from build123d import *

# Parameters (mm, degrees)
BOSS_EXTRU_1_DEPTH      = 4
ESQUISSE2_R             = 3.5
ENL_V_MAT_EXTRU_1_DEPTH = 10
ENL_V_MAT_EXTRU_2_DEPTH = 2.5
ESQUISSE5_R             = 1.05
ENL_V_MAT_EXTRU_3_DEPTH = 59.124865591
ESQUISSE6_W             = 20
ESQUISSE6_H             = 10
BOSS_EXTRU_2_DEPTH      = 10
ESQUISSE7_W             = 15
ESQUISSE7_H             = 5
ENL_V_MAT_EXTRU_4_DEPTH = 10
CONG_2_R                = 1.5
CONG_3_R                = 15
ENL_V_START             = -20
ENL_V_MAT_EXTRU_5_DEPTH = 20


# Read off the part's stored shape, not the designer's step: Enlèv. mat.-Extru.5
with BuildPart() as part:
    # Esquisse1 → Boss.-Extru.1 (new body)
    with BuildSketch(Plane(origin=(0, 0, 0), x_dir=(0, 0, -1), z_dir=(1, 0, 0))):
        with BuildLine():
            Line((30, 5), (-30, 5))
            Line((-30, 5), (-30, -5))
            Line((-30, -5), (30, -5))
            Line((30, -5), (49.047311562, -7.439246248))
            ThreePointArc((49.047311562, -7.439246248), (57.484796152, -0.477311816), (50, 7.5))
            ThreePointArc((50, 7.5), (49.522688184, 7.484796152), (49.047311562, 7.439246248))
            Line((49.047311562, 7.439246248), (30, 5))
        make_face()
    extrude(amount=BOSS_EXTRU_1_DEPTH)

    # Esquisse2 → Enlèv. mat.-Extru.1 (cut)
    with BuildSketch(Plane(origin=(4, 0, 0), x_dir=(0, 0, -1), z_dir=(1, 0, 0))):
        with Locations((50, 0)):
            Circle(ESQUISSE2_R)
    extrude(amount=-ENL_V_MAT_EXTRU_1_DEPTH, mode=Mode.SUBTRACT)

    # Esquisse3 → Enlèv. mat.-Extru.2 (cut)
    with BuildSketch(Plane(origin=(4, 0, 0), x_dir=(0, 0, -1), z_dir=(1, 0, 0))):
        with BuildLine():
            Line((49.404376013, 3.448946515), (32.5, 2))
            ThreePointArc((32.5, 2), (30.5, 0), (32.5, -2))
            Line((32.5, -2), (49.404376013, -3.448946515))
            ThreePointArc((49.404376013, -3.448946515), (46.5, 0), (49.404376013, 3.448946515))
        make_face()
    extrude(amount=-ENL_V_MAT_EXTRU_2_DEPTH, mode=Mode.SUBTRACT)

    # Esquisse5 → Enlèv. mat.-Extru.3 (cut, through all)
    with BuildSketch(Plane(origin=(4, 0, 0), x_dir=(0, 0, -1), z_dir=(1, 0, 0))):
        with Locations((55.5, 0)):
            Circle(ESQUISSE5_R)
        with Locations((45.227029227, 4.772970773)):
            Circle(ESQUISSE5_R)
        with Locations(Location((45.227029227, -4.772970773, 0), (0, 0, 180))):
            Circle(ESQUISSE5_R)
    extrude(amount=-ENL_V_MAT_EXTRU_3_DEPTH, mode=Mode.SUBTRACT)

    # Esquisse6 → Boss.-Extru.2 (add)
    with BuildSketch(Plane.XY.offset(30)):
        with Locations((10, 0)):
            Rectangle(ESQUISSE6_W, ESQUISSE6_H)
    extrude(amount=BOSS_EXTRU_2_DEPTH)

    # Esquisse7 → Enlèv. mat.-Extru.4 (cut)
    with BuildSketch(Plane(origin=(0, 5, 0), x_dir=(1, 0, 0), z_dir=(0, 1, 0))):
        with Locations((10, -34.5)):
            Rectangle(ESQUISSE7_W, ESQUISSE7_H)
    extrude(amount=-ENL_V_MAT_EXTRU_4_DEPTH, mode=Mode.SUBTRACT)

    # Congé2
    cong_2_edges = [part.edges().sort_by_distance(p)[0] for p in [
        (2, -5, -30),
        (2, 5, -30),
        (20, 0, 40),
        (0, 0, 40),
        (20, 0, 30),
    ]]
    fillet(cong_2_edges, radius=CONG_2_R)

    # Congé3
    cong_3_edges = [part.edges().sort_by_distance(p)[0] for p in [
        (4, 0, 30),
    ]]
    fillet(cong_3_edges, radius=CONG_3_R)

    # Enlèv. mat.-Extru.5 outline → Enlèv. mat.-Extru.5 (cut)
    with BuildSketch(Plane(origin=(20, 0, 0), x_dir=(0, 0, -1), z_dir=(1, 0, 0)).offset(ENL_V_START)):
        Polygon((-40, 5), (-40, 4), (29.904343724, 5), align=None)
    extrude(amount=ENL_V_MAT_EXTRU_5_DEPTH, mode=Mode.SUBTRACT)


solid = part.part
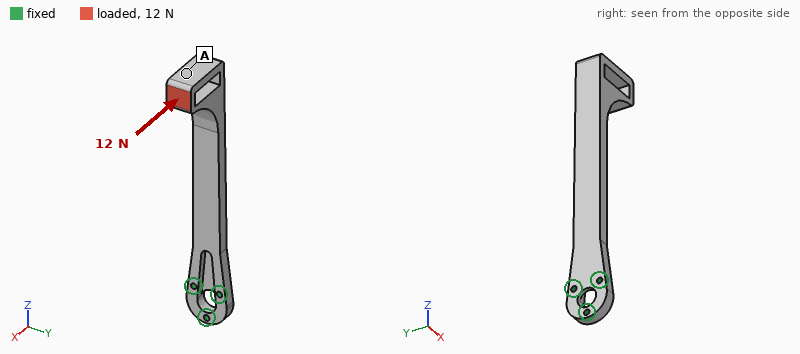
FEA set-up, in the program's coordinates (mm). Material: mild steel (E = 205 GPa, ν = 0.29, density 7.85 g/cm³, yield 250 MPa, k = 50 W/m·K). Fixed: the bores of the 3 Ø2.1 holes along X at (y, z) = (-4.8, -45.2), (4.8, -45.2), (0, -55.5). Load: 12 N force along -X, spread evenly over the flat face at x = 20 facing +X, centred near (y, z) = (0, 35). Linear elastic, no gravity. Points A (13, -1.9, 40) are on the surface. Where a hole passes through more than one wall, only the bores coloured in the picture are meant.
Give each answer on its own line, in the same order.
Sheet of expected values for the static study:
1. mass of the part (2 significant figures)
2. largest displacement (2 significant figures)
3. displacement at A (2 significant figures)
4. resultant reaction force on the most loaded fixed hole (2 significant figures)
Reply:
38 g
0.23 mm
0.22 mm
25 N
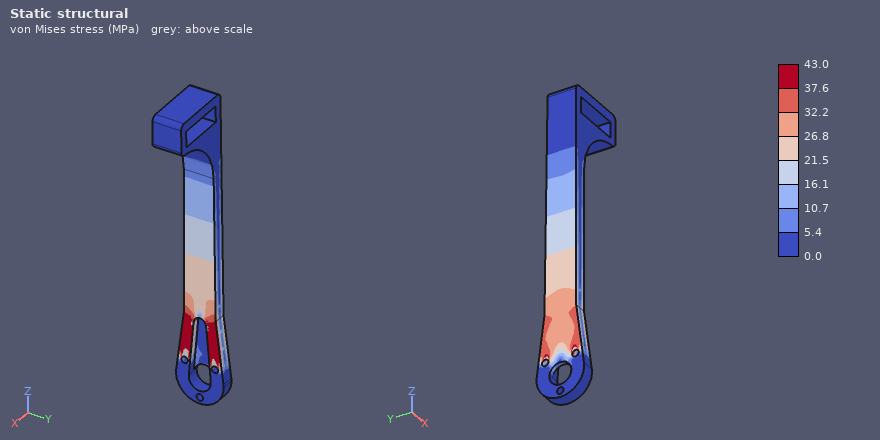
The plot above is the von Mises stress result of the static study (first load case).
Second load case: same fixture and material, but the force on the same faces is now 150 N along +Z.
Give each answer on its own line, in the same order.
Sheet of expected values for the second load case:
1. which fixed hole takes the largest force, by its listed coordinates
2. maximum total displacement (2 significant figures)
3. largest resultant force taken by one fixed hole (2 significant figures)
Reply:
(-4.8, -45.2)
0.96 mm
98 N
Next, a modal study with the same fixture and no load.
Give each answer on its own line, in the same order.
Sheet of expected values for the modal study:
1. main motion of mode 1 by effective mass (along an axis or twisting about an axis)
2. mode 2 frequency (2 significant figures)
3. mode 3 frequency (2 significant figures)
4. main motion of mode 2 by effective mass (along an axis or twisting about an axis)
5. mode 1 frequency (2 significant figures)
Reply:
along X
840 Hz
2200 Hz
along Y
310 Hz
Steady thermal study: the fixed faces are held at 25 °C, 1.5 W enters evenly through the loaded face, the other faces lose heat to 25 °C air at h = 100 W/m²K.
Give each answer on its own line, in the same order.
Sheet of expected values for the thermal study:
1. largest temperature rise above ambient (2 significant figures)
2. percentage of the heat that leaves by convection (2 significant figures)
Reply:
14 K
96 %
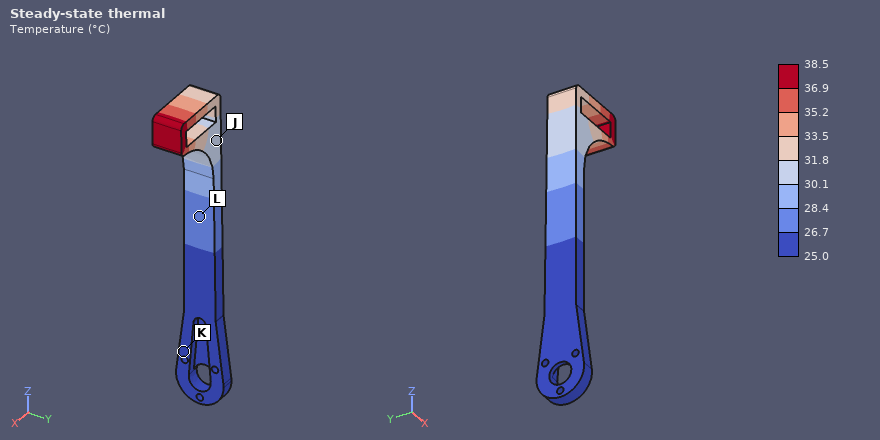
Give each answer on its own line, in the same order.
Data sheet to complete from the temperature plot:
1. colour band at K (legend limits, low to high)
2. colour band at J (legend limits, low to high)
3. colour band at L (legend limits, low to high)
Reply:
25.0 to 26.7 °C
30.1 to 31.8 °C
26.7 to 28.4 °C
